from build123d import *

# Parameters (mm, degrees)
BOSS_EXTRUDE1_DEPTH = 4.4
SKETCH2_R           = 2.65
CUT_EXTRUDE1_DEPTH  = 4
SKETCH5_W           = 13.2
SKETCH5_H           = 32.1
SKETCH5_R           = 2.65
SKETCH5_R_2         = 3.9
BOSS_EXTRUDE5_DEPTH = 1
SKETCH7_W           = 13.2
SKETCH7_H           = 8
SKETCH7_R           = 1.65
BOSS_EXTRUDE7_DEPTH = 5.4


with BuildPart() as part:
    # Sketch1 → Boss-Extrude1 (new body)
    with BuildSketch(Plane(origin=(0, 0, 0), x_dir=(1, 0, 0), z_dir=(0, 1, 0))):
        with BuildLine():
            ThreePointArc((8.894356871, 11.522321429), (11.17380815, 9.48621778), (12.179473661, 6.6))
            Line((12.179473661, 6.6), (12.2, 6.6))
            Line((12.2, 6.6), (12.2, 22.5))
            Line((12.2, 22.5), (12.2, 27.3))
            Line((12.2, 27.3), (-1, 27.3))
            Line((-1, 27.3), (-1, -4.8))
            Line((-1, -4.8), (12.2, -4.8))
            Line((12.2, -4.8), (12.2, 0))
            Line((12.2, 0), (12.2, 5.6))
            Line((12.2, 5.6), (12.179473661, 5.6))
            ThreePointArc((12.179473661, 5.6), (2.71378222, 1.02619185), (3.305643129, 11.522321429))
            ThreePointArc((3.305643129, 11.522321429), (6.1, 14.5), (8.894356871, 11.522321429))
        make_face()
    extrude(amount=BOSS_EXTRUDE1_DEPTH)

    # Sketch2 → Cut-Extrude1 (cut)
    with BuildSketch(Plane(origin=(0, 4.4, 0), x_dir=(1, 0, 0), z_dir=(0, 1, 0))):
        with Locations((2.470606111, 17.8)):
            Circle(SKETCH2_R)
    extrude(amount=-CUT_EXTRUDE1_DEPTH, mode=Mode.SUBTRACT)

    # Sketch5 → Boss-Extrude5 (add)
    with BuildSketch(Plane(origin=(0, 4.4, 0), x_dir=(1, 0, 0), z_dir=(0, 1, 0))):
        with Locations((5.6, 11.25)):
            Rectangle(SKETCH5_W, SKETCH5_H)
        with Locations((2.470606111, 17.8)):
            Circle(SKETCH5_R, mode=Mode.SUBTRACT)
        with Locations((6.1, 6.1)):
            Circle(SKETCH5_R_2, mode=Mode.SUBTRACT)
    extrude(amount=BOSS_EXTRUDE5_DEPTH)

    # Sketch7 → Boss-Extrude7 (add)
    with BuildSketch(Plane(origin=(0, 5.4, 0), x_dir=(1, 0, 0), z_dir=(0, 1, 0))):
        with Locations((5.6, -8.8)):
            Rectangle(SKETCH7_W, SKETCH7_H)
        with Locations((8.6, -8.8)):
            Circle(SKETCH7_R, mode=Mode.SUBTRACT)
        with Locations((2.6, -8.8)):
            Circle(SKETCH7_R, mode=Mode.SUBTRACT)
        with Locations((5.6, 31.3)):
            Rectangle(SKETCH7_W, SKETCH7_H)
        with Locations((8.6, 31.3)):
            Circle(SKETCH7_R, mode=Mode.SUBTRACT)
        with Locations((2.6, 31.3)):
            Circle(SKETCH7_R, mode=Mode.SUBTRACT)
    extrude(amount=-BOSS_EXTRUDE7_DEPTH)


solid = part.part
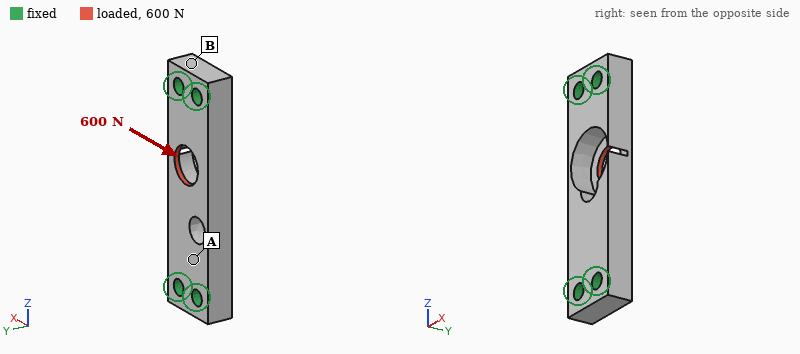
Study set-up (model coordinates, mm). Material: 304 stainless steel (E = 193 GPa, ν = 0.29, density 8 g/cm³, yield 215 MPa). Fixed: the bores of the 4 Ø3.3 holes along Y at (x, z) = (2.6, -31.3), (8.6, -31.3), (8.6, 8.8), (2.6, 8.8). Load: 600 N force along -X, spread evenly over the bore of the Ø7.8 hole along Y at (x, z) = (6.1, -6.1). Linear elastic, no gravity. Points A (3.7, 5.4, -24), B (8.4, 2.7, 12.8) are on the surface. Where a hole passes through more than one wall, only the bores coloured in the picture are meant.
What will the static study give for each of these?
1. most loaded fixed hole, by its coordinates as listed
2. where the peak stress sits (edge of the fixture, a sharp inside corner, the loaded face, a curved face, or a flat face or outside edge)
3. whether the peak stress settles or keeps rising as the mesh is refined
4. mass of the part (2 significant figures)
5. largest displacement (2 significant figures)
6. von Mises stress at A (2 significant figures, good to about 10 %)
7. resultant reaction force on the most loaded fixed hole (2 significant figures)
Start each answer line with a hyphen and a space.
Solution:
- (8.6, -31.3)
- a sharp inside corner
- keeps rising
- 20 g
- 6.9 µm
- 21 MPa
- 470 N
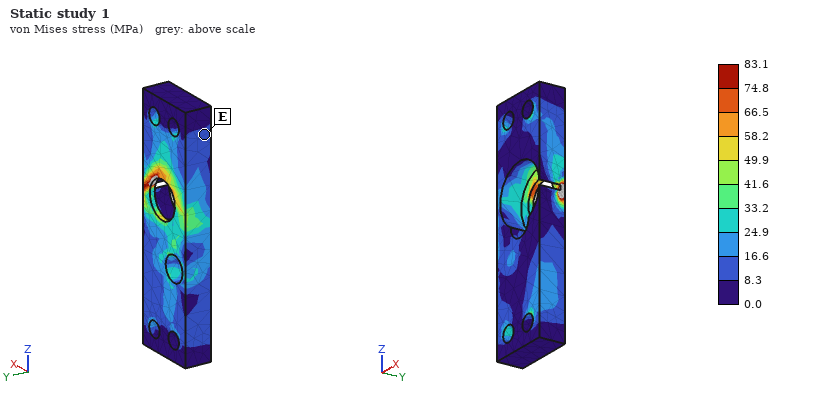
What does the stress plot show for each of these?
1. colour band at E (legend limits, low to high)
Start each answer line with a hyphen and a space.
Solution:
- 8.3 to 16.6 MPa
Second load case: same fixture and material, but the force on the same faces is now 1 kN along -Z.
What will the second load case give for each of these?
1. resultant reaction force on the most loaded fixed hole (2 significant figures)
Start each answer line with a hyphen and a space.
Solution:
- 300 N
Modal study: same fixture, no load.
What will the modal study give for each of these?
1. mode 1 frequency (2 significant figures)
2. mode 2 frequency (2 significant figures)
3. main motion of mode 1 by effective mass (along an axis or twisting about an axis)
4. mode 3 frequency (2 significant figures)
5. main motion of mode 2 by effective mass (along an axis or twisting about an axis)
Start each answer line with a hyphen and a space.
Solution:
- 17 kHz
- 25 kHz
- along Y
- 27 kHz
- along X
